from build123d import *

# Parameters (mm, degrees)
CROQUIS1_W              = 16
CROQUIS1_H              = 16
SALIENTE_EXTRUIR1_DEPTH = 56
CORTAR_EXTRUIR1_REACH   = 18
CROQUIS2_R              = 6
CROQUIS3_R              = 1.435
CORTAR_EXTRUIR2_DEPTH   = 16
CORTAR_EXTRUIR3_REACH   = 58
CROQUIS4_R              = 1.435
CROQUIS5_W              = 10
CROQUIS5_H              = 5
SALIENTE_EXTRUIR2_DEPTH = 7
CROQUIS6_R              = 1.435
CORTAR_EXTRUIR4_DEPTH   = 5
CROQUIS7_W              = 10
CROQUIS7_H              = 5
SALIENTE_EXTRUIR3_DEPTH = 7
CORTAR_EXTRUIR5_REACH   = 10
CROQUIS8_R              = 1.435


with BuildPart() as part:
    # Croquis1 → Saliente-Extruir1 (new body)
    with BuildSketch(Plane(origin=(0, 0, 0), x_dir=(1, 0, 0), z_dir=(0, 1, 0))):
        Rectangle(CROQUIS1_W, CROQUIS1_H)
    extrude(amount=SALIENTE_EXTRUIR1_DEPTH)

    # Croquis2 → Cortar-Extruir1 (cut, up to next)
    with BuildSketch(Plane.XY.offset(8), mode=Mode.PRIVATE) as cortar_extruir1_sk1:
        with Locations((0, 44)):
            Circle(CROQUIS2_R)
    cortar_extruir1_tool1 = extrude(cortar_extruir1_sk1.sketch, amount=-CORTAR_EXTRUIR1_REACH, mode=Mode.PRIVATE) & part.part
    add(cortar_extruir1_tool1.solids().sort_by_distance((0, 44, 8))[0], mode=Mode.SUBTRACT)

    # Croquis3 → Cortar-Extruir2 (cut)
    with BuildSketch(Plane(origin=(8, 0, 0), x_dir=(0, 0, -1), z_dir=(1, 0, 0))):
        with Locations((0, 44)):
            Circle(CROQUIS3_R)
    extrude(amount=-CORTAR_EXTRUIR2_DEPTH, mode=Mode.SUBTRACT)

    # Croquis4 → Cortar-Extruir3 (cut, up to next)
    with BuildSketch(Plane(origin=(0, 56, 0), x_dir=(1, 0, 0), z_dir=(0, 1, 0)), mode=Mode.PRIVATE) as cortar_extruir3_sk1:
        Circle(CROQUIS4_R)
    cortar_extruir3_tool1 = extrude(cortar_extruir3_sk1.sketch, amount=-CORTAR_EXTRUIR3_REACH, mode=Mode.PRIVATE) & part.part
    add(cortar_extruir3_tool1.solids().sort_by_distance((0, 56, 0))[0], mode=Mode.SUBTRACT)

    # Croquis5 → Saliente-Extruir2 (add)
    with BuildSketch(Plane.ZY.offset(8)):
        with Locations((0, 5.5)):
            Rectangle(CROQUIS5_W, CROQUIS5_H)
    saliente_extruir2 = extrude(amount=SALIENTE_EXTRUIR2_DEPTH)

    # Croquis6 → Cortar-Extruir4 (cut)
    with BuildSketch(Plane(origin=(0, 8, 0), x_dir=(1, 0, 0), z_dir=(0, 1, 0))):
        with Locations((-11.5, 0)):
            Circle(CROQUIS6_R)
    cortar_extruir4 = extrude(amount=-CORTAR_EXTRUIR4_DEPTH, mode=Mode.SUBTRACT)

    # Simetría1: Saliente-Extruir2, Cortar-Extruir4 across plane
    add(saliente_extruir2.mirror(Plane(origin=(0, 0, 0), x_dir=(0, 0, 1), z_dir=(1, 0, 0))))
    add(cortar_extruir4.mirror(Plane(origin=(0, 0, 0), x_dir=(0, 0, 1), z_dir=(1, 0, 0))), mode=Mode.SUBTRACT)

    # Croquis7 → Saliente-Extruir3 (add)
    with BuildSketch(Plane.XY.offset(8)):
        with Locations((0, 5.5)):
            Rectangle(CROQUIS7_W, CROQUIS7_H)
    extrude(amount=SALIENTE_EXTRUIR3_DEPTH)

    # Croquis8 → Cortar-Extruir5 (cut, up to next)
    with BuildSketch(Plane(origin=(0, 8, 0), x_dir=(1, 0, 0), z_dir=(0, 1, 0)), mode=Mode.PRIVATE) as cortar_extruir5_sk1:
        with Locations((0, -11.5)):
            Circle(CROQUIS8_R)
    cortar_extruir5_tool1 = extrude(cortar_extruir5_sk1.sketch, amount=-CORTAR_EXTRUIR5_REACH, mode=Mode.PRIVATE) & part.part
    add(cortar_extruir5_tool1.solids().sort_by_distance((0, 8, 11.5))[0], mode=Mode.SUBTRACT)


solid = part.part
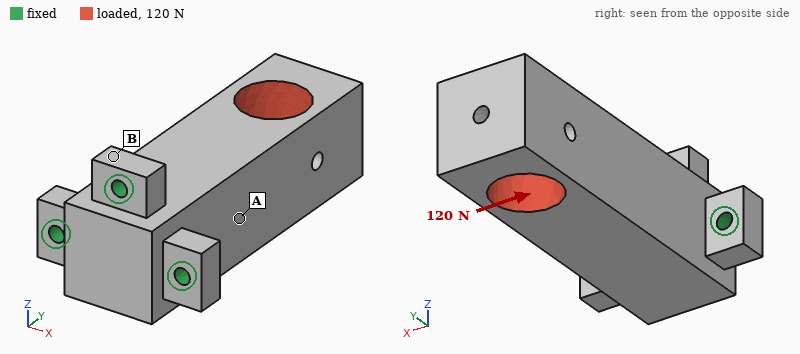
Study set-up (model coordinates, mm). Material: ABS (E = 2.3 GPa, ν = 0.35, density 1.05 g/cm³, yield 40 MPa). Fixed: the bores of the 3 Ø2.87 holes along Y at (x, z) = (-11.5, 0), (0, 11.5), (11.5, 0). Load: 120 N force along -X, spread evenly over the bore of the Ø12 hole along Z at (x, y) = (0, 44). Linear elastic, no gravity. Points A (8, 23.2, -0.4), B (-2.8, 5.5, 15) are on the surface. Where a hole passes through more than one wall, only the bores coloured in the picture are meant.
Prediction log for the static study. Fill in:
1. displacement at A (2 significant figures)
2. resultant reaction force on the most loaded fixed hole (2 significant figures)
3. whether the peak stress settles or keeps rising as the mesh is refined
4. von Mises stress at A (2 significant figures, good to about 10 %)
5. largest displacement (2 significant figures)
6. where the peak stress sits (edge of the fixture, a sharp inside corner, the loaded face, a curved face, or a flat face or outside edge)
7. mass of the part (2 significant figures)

0.13 mm
230 N
keeps rising
3.7 MPa
0.51 mm
edge of the fixture
14 g
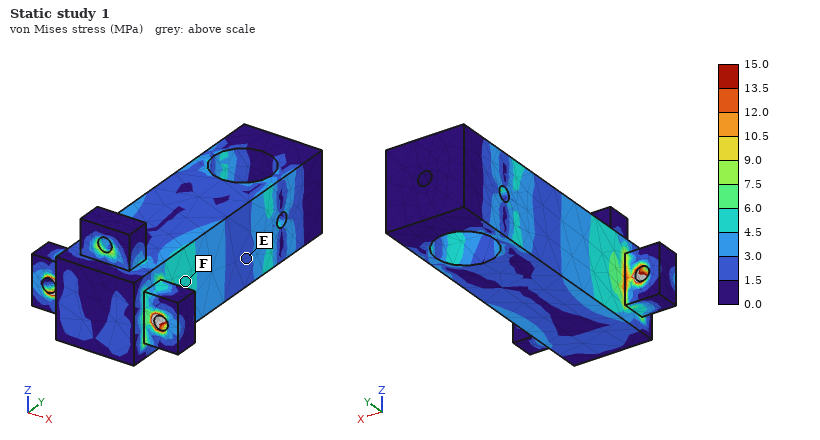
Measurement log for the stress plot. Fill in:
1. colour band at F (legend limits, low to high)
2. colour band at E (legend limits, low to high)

4.5 to 6.0 MPa
1.5 to 3.0 MPa
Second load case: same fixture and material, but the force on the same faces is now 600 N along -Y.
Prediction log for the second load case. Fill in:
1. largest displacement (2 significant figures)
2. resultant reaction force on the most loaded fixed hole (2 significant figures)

0.25 mm
260 N
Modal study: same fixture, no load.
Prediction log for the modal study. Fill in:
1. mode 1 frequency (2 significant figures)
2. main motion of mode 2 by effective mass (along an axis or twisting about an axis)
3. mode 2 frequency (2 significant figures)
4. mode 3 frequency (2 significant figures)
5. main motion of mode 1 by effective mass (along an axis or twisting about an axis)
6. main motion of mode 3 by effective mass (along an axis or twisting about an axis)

970 Hz
along X
1200 Hz
4000 Hz
along Z
twisting about Y
